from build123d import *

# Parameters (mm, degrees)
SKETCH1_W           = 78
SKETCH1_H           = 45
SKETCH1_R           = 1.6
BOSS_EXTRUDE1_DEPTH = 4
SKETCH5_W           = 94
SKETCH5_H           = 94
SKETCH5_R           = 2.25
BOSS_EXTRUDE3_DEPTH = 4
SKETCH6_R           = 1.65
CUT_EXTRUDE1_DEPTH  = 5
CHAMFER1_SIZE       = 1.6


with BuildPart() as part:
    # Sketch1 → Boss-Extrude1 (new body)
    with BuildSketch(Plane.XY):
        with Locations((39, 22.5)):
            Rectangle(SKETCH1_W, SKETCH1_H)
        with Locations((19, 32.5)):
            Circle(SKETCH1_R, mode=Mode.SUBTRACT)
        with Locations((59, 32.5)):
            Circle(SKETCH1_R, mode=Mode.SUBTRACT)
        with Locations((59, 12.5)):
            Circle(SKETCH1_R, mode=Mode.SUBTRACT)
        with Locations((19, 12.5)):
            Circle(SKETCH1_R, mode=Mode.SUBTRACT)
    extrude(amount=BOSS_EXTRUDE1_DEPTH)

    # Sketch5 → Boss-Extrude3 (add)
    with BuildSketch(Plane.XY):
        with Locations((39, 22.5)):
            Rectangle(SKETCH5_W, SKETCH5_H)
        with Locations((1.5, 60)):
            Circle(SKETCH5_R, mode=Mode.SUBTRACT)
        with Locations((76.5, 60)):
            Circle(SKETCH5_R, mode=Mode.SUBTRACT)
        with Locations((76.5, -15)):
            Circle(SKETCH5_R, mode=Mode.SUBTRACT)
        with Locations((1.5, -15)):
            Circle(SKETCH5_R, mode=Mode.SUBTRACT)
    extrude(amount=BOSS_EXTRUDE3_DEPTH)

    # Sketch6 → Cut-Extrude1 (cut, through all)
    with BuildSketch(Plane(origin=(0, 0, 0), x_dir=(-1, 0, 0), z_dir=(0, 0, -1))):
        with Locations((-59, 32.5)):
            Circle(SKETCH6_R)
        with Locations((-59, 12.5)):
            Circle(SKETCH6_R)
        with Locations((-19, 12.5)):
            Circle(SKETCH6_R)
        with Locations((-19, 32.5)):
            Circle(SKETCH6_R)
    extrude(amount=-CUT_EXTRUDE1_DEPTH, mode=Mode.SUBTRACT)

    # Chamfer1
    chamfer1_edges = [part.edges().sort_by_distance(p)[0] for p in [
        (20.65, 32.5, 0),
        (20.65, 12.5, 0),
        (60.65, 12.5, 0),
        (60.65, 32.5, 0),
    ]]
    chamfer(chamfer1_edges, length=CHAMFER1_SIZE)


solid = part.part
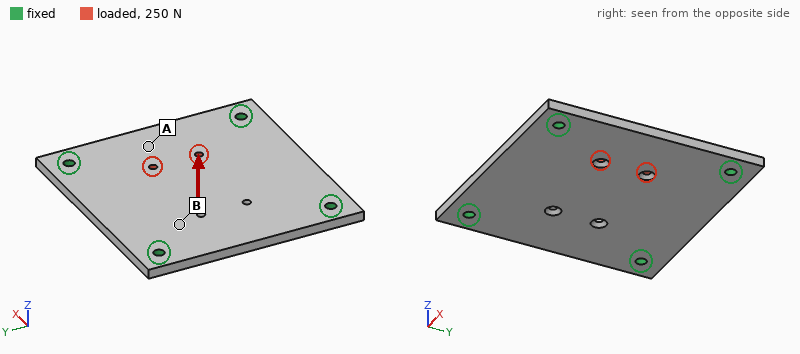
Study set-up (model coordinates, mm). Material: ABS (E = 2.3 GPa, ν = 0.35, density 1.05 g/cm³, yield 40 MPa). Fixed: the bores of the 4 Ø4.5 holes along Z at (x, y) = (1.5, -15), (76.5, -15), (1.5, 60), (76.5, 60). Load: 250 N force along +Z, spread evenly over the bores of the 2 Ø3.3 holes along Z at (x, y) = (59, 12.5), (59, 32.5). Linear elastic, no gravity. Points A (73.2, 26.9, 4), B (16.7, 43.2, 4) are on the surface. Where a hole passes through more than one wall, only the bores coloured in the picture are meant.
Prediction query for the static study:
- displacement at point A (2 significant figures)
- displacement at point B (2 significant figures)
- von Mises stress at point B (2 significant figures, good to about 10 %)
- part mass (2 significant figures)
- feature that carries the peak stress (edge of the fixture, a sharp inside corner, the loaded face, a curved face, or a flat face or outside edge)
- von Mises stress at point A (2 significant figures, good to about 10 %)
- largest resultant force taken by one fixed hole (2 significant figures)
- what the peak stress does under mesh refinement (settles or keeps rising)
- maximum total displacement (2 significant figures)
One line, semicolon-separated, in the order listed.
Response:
0.85 mm; 0.32 mm; 2.2 MPa; 37 g; edge of the fixture; 9.5 MPa; 100 N; keeps rising; 1.2 mm
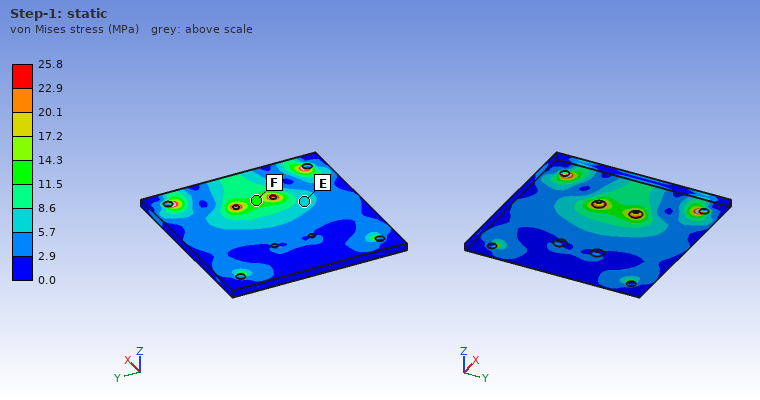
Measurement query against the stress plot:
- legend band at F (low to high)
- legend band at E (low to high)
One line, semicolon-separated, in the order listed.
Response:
11.5 to 14.3 MPa; 5.7 to 8.6 MPa
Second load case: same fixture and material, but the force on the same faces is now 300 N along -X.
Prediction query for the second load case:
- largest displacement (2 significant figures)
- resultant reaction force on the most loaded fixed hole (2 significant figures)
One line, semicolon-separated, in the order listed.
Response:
45 µm; 90 N
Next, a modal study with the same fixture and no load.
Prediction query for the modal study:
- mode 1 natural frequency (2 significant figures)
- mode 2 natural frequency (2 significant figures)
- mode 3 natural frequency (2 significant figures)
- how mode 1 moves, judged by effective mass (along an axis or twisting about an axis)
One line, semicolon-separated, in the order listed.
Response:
730 Hz; 1200 Hz; 1200 Hz; along Z
